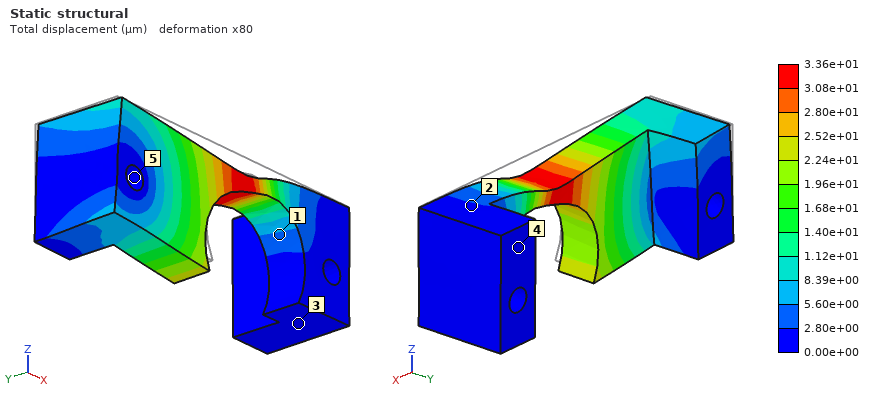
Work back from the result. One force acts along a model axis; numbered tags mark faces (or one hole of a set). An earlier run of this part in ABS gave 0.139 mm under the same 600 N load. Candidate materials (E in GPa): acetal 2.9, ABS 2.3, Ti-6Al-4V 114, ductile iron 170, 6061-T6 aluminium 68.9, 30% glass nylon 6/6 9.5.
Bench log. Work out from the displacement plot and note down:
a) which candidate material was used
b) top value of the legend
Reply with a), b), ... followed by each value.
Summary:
a) 30% glass nylon 6/6
b) 3.36e+01 µm
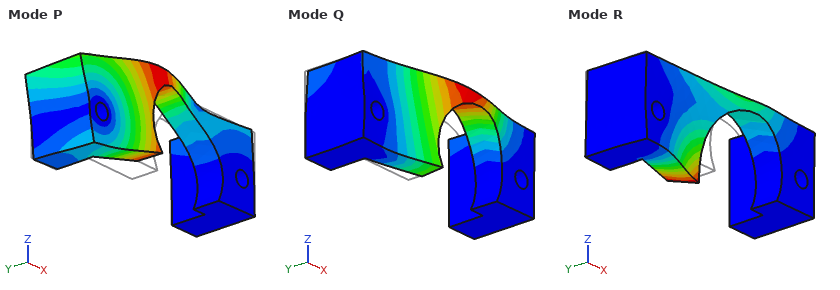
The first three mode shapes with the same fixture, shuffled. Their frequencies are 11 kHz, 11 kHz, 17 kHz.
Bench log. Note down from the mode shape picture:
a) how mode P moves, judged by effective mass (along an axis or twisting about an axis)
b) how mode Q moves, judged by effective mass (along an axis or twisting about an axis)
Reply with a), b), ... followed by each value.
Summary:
a) along Z
b) along Y
